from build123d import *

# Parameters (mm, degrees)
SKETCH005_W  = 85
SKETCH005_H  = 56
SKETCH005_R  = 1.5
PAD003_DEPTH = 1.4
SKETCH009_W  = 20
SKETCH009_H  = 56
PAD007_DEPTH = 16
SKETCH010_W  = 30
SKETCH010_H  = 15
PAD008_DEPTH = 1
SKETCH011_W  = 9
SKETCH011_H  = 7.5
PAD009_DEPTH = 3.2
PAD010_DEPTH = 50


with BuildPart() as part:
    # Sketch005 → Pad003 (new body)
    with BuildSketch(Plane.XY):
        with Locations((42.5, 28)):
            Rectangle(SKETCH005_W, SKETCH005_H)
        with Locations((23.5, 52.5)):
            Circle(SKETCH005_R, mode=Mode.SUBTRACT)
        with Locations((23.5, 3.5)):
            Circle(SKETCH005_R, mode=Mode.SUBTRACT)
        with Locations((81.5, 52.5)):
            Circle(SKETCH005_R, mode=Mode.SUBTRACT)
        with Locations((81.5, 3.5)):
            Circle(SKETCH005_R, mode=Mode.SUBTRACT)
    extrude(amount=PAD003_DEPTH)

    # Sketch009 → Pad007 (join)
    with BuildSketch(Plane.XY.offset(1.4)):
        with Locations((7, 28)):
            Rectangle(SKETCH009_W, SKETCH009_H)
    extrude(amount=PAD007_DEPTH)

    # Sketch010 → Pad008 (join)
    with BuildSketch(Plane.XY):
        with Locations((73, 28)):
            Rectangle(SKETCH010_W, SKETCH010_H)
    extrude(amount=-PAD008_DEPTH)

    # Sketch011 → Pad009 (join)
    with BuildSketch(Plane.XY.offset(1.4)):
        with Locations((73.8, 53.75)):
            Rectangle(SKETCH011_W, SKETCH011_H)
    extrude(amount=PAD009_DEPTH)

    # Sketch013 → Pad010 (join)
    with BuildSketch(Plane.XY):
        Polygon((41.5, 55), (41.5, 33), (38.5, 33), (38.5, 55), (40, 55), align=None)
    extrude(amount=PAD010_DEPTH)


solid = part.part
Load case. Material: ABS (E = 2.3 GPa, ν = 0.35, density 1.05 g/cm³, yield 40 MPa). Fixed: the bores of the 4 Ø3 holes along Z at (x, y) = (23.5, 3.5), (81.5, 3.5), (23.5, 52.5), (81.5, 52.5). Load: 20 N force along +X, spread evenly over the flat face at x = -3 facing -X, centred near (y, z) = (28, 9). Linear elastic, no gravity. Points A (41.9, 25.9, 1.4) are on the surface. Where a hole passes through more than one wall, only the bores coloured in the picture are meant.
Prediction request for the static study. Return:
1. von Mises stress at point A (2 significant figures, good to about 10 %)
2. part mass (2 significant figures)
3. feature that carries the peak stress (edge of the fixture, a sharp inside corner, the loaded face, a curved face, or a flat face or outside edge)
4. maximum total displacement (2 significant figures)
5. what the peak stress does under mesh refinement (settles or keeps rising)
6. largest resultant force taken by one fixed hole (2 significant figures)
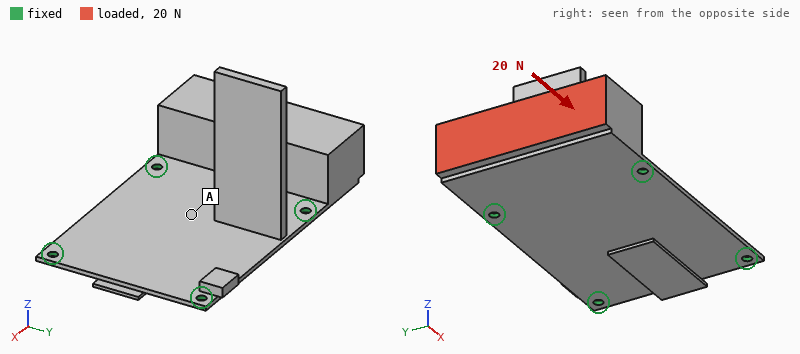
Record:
1.6 MPa
30 g
edge of the fixture
1.4 mm
keeps rising
8.4 N
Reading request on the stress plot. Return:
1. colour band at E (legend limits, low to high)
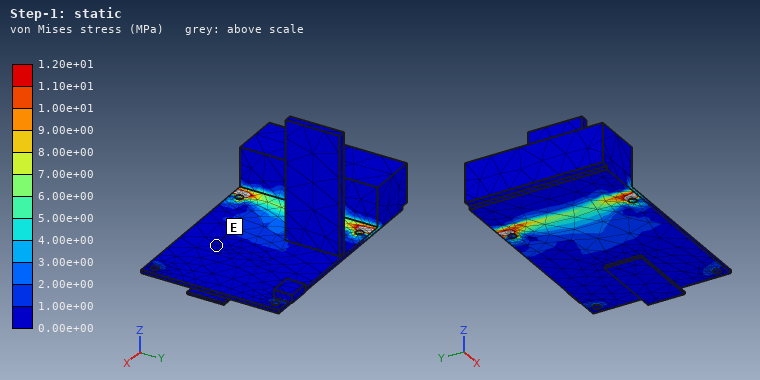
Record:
0.00e+00 to 1.00e+00 MPa
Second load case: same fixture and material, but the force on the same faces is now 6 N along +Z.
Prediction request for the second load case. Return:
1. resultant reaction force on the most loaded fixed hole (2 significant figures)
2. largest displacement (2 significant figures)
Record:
3.4 N
1.1 mm
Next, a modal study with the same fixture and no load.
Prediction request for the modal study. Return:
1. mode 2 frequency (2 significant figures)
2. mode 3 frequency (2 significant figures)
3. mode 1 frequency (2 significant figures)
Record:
170 Hz
250 Hz
120 Hz
